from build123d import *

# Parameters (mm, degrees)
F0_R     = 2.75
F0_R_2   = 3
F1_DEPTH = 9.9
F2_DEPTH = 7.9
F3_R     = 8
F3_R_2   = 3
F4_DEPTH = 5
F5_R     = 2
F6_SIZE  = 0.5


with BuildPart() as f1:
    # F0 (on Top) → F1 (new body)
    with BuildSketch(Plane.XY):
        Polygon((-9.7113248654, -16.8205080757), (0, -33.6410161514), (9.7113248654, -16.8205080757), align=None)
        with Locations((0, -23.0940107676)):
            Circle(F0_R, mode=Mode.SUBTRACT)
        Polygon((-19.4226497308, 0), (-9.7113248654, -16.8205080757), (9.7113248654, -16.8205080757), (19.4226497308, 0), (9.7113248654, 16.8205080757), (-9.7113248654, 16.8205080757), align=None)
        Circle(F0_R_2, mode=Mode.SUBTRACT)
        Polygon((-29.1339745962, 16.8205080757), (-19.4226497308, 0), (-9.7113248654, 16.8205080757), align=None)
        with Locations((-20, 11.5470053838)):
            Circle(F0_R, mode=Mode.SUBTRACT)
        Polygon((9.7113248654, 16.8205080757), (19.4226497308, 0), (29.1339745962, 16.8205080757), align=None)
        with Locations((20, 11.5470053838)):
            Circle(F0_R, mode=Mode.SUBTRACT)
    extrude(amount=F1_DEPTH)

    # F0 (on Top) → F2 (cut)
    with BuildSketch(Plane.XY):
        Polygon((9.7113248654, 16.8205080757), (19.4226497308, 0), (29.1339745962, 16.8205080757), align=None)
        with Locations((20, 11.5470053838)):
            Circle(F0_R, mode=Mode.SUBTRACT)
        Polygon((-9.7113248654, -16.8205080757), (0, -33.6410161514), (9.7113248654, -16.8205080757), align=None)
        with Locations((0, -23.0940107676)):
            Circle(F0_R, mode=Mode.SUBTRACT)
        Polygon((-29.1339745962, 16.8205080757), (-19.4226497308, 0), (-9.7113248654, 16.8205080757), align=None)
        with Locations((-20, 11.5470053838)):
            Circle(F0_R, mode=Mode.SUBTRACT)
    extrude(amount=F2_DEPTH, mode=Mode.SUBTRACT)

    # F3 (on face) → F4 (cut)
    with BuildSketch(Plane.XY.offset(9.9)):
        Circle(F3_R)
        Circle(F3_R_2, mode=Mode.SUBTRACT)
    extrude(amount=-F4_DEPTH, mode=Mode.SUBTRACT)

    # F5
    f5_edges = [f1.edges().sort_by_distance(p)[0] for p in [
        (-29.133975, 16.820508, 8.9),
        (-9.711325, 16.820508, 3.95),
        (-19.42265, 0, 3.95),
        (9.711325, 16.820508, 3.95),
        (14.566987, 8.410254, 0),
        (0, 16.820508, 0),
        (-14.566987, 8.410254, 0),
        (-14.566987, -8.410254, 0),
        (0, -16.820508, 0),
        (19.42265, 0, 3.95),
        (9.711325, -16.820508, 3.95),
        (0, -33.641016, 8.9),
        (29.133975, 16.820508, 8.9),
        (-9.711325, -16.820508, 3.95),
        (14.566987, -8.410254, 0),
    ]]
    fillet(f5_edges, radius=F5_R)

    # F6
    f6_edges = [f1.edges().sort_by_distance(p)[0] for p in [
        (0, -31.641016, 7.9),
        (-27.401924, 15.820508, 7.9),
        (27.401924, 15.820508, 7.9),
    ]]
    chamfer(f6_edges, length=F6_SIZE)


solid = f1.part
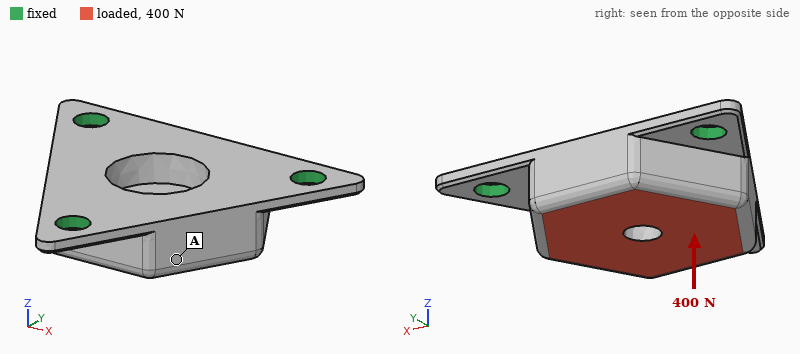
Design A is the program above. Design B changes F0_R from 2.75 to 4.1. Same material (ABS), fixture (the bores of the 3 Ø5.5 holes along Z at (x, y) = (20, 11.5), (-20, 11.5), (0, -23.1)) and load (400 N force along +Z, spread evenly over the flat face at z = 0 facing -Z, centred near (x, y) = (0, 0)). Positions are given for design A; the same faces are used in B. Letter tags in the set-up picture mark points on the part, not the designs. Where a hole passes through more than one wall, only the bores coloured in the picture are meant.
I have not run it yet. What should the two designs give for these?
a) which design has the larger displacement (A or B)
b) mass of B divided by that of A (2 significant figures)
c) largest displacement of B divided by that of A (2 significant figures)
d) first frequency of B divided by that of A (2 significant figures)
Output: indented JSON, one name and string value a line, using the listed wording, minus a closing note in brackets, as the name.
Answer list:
{
  "which design has the larger displacement": "A",
  "mass of B divided by that of A": "0.98",
  "largest displacement of B divided by that of A": "0.56",
  "first frequency of B divided by that of A": "1.4"
}
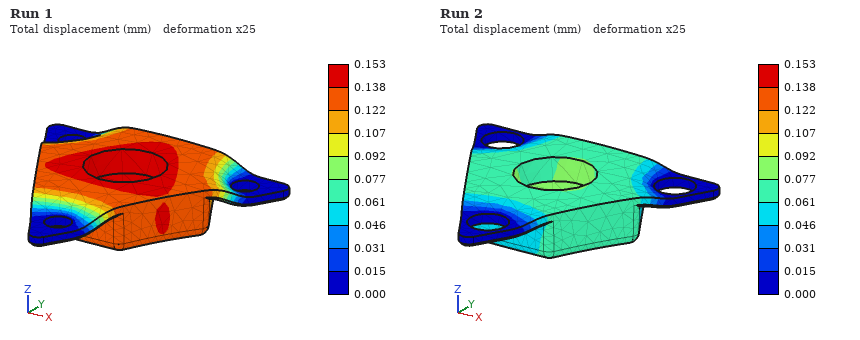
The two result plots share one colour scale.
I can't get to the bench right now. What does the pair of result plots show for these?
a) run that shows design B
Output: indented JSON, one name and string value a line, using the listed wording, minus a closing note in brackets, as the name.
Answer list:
{
  "run that shows design B": "Run 2"
}
